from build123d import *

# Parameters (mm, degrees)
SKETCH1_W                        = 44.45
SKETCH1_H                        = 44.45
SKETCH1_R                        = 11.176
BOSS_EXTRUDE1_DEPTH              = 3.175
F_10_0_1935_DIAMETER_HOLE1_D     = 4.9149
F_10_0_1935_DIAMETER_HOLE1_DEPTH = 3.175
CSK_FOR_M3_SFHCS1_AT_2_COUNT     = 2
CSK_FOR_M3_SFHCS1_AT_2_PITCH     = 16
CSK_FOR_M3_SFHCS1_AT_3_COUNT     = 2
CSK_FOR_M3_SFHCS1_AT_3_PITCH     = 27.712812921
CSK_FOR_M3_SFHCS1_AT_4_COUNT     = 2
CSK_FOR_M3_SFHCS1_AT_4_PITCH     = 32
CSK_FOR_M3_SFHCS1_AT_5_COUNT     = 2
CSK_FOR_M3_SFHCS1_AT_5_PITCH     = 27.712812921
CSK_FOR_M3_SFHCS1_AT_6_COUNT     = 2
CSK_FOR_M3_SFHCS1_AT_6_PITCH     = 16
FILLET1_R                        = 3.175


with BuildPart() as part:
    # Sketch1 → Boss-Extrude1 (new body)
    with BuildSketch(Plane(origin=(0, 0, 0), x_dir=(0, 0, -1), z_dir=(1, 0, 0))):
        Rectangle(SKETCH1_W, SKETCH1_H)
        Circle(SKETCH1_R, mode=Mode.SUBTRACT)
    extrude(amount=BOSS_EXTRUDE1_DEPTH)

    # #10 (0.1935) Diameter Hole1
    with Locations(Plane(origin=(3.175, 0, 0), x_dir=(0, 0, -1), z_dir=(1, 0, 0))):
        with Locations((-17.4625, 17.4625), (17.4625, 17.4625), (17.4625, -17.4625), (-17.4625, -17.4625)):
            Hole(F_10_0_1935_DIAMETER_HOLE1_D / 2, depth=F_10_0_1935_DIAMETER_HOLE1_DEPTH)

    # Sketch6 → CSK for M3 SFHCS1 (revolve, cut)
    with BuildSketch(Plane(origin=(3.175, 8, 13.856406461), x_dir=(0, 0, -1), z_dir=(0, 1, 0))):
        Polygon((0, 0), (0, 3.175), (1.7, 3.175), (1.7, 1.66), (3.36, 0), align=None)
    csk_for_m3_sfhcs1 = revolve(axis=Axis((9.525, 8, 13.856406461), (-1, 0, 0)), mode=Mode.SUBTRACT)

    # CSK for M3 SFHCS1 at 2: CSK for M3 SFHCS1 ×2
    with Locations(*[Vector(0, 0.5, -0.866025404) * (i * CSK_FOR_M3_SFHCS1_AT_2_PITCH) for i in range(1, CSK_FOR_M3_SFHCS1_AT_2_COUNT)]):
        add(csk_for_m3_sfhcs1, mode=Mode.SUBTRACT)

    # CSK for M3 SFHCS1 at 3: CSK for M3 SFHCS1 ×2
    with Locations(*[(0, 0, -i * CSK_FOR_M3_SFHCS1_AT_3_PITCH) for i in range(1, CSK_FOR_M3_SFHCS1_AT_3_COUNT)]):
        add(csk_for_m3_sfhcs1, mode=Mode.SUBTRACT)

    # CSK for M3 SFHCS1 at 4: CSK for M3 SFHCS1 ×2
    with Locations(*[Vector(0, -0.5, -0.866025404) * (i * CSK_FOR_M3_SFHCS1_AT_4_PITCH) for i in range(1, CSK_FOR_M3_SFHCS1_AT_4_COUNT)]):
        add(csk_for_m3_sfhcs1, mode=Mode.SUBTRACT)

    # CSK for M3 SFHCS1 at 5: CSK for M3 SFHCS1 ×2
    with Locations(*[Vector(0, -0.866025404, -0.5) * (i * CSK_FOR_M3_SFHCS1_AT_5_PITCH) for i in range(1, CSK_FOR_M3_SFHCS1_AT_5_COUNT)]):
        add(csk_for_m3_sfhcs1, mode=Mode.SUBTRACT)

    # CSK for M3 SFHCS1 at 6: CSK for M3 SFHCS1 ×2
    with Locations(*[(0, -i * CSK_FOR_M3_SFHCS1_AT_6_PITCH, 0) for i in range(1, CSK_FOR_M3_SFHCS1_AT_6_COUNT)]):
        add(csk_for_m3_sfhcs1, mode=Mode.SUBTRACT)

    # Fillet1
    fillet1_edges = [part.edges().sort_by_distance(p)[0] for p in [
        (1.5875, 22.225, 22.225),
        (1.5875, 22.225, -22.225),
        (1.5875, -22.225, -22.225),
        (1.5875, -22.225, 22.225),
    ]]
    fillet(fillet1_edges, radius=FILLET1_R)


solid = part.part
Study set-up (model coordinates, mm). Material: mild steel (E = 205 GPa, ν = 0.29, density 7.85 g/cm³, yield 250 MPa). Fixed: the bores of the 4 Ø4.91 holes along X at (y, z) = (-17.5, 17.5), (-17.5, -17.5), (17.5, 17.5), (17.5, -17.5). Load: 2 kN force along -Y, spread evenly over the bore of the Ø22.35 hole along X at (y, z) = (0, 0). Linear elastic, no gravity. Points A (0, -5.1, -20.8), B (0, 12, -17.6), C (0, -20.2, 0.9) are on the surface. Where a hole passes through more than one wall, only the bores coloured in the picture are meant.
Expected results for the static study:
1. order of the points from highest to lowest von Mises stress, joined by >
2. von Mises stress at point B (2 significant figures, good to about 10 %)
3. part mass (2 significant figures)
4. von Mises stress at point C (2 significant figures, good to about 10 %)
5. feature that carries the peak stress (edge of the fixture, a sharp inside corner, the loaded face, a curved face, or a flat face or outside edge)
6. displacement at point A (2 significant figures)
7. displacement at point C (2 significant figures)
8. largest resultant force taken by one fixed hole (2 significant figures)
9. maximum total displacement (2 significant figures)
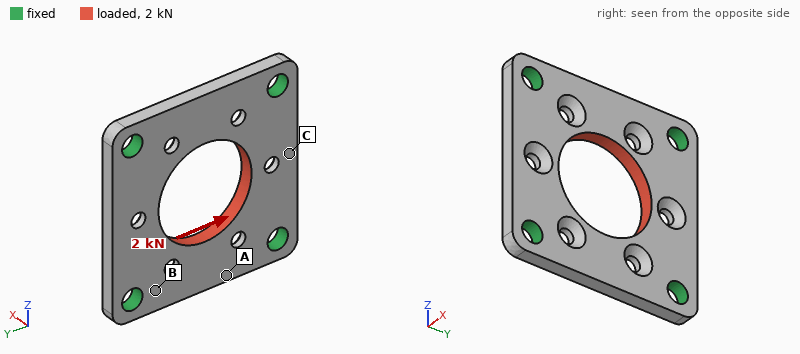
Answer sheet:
B > C > A
14 MPa
35 g
9.3 MPa
a curved face
0.43 µm
1.8 µm
530 N
2.3 µm
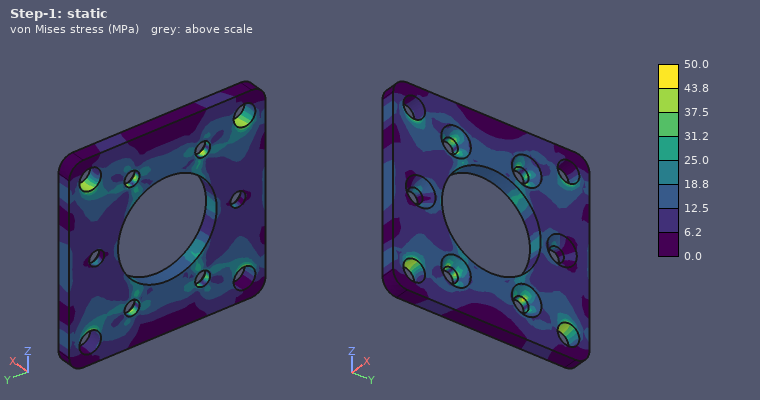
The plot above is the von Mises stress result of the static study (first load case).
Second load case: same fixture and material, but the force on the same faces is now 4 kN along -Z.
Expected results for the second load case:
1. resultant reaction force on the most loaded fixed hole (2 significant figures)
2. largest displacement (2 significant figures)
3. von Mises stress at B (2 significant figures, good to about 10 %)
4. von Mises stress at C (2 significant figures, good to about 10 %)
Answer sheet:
1.0 kN
4.8 µm
22 MPa
22 MPa
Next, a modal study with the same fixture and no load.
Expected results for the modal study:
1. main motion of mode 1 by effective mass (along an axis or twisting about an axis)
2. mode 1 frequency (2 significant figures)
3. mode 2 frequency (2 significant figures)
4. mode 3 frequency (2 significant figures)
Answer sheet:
along X
14 kHz
16 kHz
16 kHz
